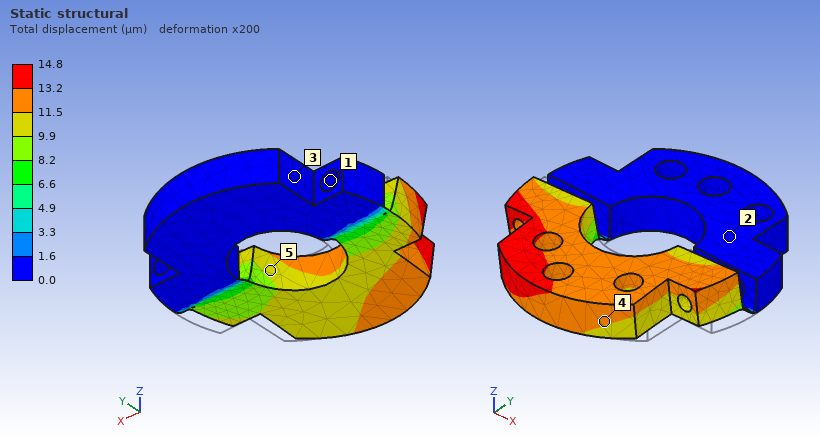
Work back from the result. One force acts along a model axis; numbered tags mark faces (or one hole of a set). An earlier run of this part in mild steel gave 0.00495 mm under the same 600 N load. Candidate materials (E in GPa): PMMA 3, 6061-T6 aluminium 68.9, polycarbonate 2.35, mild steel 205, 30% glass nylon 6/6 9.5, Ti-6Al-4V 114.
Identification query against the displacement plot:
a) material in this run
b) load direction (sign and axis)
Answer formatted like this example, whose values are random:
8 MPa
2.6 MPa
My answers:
6061-T6 aluminium
-X
